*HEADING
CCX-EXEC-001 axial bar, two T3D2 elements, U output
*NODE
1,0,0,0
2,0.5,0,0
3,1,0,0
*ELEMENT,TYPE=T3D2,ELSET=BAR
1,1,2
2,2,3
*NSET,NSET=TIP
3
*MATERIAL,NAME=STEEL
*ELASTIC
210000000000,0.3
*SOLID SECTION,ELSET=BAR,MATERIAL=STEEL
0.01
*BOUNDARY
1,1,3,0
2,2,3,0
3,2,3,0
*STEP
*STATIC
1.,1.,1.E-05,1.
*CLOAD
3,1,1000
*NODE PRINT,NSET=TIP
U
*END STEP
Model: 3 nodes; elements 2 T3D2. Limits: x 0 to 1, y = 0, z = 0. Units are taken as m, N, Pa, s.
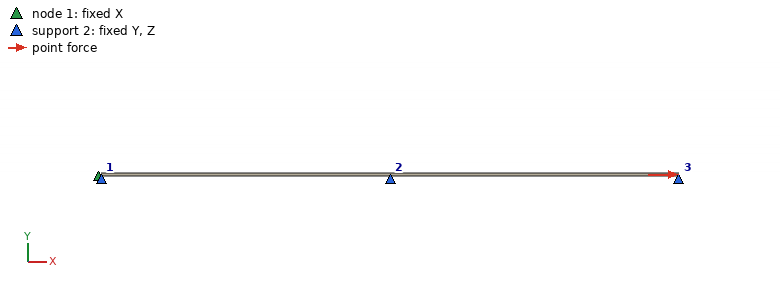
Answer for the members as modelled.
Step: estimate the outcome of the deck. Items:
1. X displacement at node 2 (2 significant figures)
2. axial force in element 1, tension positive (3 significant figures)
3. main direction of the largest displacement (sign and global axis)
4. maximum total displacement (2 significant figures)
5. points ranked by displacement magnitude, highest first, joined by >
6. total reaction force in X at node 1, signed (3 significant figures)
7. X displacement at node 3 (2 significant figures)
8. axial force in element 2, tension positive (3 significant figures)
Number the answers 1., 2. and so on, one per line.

1. 2.4e-07 m
2. 1000 N
3. +X
4. 4.8e-07 m
5. node 3 > node 2 > node 1
6. -1000 N
7. 4.8e-07 m
8. 1000 N
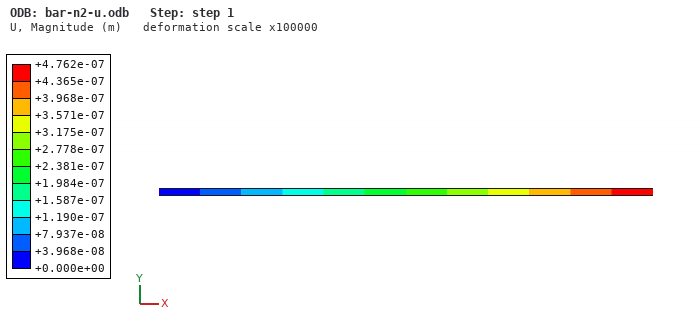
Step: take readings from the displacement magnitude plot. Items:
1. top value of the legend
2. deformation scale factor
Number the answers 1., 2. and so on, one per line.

1. +4.762e-07 m
2. 100000
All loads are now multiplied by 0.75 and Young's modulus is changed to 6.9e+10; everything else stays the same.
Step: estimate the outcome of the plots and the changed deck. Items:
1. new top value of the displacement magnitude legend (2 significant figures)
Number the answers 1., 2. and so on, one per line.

1. 1.1e-06 m
